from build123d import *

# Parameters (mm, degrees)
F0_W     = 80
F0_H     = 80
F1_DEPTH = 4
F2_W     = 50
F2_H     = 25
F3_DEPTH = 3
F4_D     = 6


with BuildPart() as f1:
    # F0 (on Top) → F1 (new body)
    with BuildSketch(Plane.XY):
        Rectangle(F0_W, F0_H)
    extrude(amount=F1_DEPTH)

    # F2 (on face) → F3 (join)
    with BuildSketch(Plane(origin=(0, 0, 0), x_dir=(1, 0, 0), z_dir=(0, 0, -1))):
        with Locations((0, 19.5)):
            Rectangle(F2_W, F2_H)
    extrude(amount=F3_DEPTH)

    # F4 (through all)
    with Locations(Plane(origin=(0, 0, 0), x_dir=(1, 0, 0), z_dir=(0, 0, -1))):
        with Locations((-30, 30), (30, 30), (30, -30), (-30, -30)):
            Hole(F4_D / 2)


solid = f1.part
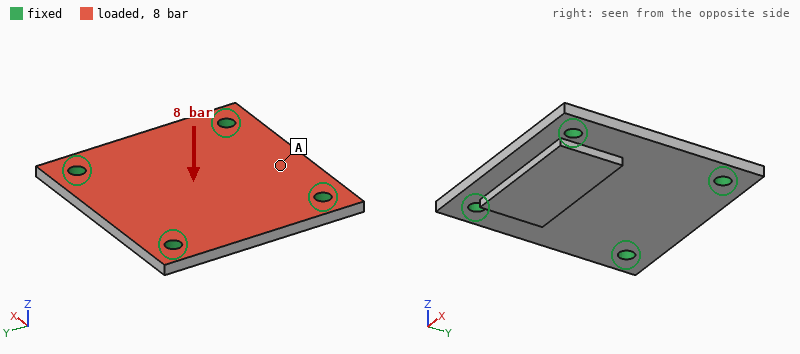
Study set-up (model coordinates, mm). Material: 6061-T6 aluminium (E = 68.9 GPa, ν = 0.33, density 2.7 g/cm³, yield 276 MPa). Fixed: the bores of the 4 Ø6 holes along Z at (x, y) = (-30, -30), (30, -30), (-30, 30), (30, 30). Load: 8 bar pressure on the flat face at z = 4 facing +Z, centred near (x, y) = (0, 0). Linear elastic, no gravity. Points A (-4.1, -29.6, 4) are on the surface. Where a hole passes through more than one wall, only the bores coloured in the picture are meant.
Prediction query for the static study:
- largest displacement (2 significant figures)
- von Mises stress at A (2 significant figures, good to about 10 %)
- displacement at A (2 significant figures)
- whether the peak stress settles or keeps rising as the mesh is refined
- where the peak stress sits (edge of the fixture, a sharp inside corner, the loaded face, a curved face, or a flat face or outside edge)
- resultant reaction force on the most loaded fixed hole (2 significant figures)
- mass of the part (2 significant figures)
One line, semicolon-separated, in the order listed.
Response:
0.13 mm; 26 MPa; 0.041 mm; keeps rising; edge of the fixture; 1.4 kN; 78 g
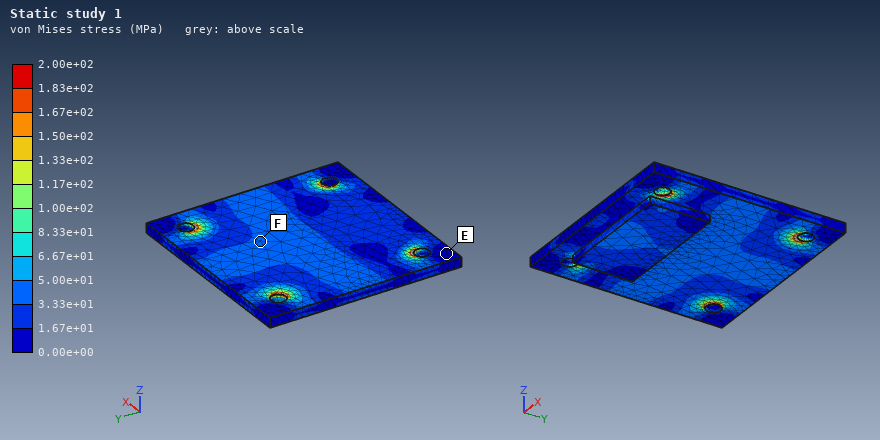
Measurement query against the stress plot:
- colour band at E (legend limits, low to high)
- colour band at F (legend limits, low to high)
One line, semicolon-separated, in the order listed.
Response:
0.00e+00 to 1.67e+01 MPa; 3.33e+01 to 5.00e+01 MPa
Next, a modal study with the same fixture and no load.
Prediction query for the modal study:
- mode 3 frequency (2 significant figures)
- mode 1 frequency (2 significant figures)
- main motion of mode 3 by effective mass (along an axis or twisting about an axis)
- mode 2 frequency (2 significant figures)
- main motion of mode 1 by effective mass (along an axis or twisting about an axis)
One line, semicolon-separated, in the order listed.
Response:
7200 Hz; 4400 Hz; twisting about Y; 6800 Hz; along Z
